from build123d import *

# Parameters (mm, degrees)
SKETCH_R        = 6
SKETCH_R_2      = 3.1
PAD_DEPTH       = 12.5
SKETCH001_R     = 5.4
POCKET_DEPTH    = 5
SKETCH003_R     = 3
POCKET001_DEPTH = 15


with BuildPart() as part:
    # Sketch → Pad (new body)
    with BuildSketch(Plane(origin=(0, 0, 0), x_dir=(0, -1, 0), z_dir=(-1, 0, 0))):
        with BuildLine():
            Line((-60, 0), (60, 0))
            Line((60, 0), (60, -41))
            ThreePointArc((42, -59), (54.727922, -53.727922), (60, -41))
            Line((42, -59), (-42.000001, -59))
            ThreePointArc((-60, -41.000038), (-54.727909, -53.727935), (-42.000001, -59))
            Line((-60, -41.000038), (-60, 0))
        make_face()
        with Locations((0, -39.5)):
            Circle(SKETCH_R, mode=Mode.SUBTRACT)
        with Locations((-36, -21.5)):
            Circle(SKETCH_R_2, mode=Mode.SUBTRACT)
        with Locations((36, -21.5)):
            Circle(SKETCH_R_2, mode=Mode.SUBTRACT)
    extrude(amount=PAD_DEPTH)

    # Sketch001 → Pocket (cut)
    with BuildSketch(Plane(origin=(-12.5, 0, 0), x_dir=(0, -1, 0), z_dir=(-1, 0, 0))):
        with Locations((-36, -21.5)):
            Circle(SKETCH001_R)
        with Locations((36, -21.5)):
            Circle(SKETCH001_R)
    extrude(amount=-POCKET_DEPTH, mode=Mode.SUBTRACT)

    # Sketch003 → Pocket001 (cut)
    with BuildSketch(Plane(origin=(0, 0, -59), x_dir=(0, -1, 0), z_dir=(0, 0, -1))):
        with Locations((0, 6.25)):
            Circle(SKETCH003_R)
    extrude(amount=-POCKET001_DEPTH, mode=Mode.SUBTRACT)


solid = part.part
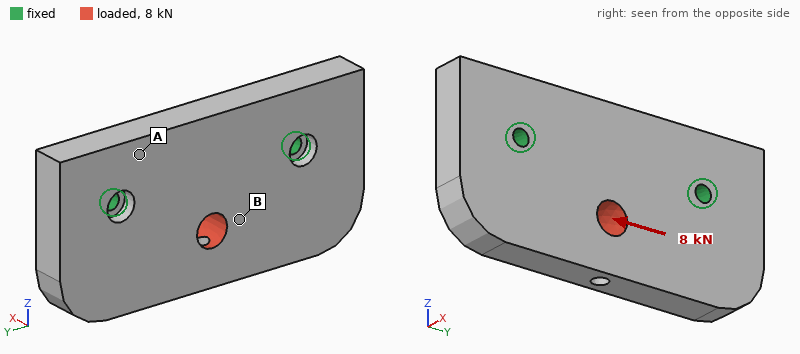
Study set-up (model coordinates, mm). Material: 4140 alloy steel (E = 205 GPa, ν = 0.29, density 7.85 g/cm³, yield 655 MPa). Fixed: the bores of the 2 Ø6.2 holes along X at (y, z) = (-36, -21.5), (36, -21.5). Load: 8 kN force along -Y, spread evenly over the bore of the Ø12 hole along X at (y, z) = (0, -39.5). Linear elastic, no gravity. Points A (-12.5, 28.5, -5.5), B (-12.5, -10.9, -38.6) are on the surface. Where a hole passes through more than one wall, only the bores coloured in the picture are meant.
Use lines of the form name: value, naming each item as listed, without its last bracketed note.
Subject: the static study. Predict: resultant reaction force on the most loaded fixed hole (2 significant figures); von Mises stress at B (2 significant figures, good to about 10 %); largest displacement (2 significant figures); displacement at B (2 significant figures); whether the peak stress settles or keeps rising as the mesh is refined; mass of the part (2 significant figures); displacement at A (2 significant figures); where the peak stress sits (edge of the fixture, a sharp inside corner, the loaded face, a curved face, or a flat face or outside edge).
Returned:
resultant reaction force on the most loaded fixed hole: 4.4 kN
von Mises stress at B: 19 MPa
largest displacement: 4.2 µm
displacement at B: 3.0 µm
whether the peak stress settles or keeps rising as the mesh is refined: keeps rising
mass of the part: 660 g
displacement at A: 0.95 µm
where the peak stress sits: edge of the fixture
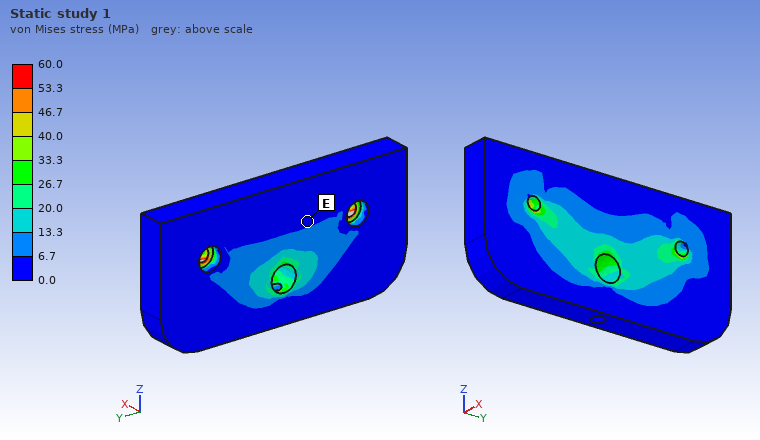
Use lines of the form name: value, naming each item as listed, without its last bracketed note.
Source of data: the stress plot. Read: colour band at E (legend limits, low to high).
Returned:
colour band at E: 0.0 to 6.7 MPa
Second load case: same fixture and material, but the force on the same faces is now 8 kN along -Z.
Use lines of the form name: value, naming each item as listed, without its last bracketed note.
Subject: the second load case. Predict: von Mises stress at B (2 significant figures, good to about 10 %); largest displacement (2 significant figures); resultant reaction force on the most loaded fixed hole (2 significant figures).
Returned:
von Mises stress at B: 14 MPa
largest displacement: 9.7 µm
resultant reaction force on the most loaded fixed hole: 4.1 kN
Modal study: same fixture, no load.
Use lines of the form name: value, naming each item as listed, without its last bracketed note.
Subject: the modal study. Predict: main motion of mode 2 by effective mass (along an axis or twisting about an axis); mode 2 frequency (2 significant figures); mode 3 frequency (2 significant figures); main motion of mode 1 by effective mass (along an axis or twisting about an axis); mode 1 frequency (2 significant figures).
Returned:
main motion of mode 2 by effective mass: twisting about Z
mode 2 frequency: 5900 Hz
mode 3 frequency: 6400 Hz
main motion of mode 1 by effective mass: along X
mode 1 frequency: 3400 Hz
